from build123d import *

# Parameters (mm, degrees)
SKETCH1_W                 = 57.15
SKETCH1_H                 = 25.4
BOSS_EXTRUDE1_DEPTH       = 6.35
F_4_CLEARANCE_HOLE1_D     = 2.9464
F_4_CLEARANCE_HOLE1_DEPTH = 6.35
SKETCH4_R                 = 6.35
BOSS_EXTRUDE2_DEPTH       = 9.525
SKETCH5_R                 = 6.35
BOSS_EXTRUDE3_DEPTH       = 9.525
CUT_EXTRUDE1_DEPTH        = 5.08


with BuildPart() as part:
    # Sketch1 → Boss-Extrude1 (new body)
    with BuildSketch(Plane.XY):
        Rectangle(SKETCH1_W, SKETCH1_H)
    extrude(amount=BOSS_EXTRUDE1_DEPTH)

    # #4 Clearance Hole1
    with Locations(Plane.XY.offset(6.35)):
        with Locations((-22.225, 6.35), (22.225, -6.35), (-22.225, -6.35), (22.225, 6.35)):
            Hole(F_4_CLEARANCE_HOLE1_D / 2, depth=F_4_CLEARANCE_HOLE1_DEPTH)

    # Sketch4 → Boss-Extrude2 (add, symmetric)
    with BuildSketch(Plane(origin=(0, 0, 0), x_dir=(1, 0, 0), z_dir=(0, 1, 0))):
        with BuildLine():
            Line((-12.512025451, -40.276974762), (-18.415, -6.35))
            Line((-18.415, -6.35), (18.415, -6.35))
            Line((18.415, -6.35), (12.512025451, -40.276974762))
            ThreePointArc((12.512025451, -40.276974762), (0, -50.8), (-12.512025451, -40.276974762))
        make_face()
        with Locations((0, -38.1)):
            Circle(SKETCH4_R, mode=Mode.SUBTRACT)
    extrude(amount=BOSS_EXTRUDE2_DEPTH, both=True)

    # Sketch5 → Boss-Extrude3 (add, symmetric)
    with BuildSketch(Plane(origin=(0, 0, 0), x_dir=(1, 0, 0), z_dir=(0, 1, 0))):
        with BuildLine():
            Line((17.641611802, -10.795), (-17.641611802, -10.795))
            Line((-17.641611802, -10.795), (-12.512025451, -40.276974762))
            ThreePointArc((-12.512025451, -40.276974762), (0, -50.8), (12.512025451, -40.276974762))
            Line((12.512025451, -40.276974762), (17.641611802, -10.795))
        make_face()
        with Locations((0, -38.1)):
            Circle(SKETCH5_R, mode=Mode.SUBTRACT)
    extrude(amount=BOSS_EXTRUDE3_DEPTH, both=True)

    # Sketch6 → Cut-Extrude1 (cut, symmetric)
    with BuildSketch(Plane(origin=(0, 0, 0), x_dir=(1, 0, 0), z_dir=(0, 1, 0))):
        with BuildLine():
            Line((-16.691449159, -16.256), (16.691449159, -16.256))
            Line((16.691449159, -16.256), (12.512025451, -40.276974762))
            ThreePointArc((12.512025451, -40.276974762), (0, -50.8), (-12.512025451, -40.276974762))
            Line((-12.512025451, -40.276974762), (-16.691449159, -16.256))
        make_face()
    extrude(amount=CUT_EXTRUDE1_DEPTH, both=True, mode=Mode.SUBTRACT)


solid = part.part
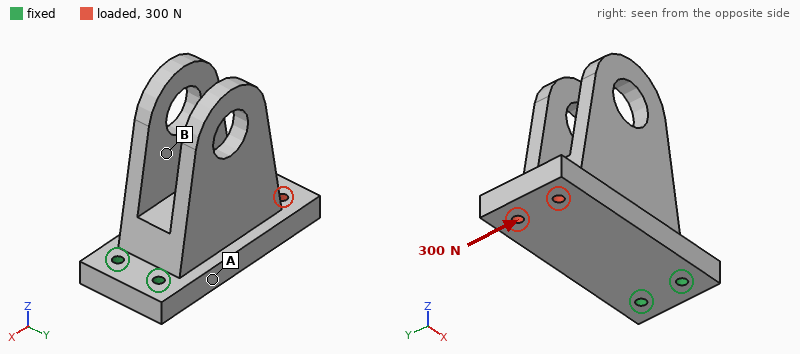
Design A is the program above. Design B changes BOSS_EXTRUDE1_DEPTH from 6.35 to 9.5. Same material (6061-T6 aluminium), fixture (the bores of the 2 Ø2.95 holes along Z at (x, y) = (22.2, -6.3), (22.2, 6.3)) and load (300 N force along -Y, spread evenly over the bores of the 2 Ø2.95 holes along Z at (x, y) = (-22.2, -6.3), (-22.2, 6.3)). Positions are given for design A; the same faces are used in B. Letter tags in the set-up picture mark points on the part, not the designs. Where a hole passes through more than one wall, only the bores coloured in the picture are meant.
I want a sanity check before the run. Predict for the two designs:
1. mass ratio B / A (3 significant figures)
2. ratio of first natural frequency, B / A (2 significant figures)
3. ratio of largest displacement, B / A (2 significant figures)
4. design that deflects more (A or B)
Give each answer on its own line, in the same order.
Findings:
1.10
1.6
0.70
A
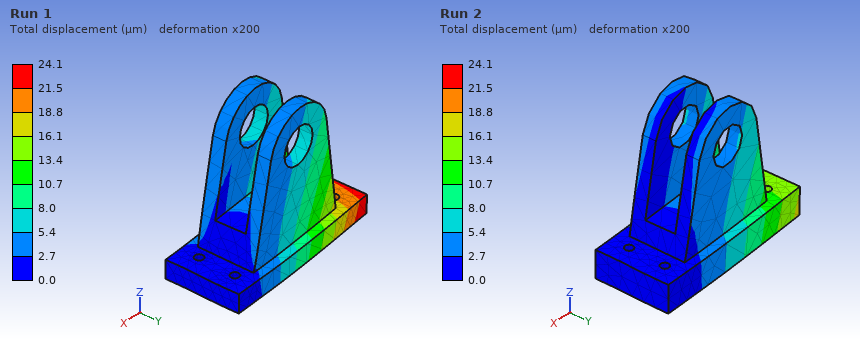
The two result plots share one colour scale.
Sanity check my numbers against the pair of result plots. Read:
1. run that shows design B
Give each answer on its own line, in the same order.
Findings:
Run 2
